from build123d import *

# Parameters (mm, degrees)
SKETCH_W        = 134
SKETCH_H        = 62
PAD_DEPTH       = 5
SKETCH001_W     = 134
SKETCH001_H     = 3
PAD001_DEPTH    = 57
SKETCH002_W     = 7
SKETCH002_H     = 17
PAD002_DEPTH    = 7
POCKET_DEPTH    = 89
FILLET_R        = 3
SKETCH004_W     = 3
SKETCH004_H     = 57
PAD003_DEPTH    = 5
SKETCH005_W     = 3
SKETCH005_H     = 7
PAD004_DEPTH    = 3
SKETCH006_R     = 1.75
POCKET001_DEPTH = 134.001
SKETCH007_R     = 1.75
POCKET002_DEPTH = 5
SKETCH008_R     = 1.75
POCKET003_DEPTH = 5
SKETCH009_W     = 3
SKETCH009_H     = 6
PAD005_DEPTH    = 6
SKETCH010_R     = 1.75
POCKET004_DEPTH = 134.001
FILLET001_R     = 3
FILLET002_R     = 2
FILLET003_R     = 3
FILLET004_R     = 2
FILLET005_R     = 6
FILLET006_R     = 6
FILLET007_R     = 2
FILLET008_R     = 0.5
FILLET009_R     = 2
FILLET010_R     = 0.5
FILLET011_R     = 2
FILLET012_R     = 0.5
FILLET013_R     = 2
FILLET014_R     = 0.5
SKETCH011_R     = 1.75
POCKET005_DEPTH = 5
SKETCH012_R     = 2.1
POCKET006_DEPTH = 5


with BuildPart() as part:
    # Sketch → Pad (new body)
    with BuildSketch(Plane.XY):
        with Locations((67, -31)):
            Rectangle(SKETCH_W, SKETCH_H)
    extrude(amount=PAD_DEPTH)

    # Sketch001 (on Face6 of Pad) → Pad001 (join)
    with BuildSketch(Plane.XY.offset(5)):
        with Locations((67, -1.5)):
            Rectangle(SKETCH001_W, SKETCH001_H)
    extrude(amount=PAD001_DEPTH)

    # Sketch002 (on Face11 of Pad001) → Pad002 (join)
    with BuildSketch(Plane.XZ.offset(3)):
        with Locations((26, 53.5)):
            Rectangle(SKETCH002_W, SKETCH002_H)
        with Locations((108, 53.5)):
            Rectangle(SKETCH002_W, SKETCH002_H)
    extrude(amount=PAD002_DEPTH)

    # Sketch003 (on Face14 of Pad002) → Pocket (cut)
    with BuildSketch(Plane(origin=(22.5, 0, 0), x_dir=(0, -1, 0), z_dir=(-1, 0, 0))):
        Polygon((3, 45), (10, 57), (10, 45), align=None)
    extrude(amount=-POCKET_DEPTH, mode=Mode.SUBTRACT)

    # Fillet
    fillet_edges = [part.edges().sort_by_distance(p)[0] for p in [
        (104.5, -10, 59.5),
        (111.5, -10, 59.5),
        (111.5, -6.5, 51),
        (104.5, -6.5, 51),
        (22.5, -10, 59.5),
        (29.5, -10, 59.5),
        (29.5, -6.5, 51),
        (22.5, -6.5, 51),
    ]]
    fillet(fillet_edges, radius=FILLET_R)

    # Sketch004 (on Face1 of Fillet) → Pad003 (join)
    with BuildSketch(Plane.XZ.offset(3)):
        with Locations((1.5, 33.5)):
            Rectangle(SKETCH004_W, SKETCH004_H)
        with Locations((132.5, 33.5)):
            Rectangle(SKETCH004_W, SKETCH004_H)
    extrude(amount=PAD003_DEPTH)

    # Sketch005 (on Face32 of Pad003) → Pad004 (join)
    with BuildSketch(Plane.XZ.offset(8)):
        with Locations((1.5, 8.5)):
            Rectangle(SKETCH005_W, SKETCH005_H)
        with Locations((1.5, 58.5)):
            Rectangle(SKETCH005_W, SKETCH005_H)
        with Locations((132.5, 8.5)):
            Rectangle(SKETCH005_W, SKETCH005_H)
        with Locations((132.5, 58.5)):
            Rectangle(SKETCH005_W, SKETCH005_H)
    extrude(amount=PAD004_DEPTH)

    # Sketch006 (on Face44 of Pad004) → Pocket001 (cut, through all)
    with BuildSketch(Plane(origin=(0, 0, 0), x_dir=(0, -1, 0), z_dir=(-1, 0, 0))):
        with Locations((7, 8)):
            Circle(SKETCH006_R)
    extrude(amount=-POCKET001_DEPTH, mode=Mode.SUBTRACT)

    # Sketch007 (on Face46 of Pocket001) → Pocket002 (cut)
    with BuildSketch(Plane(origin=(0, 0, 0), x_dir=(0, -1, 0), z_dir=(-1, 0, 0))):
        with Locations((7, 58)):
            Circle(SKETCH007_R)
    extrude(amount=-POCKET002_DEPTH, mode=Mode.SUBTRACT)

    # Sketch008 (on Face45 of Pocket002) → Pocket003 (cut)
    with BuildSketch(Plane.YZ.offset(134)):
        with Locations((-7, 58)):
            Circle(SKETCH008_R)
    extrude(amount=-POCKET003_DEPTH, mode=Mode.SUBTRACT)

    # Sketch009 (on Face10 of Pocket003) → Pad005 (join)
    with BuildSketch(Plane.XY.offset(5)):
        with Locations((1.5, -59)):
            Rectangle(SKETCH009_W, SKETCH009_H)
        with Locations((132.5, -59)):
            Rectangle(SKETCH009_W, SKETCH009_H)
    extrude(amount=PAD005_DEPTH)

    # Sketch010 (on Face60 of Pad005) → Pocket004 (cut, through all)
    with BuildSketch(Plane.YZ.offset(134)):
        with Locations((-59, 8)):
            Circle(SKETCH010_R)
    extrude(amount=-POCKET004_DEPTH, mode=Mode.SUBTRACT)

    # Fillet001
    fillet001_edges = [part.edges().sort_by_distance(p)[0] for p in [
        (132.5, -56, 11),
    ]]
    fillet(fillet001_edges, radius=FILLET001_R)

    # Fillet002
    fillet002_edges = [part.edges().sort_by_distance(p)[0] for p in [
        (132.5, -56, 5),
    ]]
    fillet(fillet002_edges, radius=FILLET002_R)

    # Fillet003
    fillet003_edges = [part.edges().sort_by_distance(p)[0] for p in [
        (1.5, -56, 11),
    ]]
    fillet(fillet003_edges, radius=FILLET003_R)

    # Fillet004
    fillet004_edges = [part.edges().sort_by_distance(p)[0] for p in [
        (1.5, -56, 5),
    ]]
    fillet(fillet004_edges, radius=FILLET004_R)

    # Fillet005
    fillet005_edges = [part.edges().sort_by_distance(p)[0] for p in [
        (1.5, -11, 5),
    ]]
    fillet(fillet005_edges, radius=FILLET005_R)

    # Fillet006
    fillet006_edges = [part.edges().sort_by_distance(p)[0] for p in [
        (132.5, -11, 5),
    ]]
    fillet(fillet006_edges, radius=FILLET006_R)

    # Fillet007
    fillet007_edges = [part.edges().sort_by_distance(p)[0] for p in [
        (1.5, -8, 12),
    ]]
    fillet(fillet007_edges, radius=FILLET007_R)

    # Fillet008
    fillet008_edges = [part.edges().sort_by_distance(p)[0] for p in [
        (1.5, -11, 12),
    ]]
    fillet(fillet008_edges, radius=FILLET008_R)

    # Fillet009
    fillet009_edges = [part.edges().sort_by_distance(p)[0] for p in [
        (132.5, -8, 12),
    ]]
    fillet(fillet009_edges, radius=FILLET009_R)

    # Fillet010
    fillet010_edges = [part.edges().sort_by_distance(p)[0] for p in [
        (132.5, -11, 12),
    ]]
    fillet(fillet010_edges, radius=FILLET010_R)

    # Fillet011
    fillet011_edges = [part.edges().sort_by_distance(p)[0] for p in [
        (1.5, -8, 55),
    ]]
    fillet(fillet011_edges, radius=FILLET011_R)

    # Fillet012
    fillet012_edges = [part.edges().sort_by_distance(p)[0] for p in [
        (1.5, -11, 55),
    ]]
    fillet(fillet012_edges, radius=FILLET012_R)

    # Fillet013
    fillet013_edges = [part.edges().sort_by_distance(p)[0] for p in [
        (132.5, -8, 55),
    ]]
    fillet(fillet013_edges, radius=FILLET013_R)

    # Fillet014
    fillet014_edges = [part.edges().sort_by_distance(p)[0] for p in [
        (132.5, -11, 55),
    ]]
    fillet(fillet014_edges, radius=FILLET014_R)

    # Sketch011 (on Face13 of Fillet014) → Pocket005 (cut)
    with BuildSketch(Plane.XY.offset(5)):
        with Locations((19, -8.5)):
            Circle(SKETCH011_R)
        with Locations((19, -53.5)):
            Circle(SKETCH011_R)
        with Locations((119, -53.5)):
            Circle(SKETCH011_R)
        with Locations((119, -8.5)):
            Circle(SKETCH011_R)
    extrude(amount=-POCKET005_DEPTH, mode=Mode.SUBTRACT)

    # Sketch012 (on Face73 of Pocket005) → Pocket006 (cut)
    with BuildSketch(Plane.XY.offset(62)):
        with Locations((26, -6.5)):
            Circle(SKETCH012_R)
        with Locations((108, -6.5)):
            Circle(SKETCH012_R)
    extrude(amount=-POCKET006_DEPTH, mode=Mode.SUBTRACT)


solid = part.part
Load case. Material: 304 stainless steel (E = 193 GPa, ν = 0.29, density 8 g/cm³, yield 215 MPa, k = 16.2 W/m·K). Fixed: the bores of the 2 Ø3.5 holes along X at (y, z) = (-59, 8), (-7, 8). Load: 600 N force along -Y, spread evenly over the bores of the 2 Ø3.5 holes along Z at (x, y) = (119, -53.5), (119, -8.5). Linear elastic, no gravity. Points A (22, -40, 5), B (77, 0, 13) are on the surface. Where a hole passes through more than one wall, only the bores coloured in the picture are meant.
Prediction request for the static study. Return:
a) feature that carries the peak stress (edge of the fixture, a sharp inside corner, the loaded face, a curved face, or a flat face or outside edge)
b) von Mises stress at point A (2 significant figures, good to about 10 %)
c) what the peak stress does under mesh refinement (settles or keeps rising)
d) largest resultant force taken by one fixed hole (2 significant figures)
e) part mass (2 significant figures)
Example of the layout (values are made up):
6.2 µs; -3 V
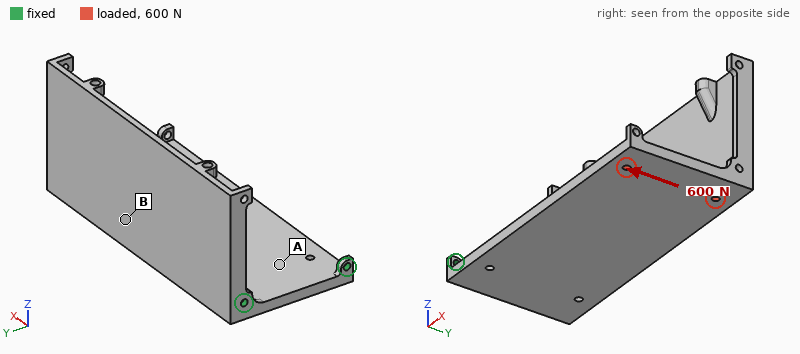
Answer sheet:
edge of the fixture; 16 MPa; keeps rising; 1.4 kN; 540 g
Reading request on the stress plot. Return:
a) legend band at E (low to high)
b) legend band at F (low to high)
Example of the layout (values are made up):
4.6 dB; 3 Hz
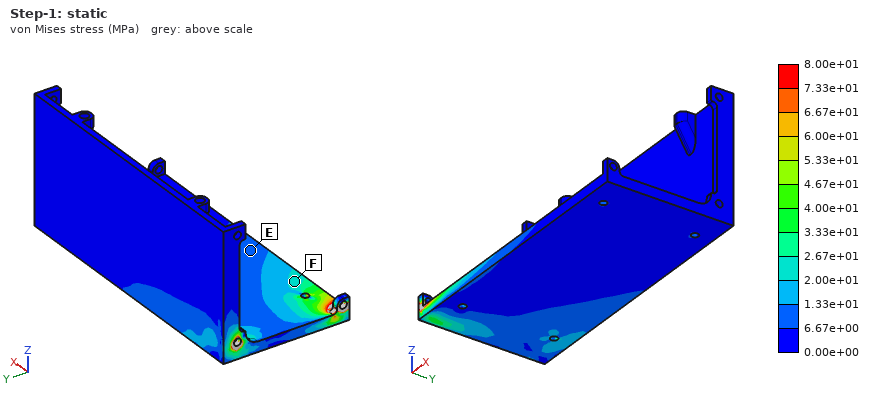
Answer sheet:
6.67e+00 to 1.33e+01 MPa; 2.00e+01 to 2.67e+01 MPa
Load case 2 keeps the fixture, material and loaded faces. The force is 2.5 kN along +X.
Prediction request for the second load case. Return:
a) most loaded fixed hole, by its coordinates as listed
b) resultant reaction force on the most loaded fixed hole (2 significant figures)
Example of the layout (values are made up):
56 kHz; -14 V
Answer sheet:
(-7, 8); 1.4 kN
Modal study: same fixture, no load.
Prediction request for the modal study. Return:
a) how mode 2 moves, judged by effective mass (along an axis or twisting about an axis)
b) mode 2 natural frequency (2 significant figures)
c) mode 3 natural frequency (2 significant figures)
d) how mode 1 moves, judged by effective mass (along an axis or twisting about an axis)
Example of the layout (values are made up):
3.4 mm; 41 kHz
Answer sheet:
along Y; 440 Hz; 1100 Hz; along Z
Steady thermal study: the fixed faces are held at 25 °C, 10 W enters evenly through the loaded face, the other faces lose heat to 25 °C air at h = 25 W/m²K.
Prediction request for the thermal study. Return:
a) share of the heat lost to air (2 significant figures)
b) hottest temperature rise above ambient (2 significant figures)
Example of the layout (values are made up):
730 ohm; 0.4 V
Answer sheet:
97 %; 62 K
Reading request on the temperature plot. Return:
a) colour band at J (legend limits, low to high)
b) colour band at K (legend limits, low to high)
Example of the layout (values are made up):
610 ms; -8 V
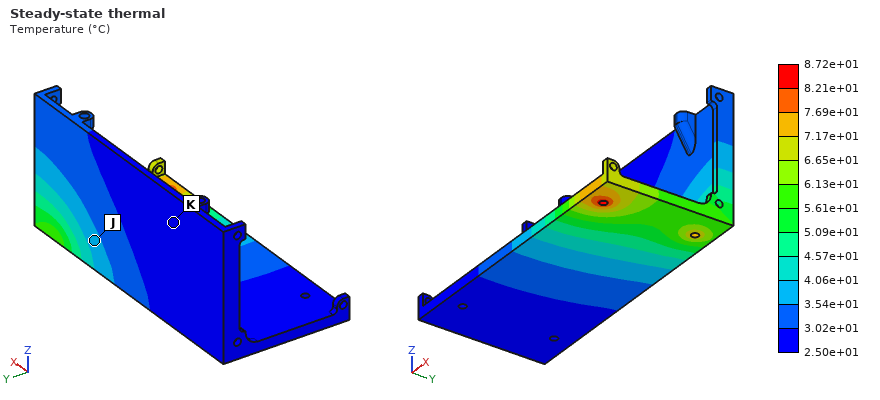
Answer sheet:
3.54e+01 to 4.06e+01 °C; 2.50e+01 to 3.02e+01 °C
